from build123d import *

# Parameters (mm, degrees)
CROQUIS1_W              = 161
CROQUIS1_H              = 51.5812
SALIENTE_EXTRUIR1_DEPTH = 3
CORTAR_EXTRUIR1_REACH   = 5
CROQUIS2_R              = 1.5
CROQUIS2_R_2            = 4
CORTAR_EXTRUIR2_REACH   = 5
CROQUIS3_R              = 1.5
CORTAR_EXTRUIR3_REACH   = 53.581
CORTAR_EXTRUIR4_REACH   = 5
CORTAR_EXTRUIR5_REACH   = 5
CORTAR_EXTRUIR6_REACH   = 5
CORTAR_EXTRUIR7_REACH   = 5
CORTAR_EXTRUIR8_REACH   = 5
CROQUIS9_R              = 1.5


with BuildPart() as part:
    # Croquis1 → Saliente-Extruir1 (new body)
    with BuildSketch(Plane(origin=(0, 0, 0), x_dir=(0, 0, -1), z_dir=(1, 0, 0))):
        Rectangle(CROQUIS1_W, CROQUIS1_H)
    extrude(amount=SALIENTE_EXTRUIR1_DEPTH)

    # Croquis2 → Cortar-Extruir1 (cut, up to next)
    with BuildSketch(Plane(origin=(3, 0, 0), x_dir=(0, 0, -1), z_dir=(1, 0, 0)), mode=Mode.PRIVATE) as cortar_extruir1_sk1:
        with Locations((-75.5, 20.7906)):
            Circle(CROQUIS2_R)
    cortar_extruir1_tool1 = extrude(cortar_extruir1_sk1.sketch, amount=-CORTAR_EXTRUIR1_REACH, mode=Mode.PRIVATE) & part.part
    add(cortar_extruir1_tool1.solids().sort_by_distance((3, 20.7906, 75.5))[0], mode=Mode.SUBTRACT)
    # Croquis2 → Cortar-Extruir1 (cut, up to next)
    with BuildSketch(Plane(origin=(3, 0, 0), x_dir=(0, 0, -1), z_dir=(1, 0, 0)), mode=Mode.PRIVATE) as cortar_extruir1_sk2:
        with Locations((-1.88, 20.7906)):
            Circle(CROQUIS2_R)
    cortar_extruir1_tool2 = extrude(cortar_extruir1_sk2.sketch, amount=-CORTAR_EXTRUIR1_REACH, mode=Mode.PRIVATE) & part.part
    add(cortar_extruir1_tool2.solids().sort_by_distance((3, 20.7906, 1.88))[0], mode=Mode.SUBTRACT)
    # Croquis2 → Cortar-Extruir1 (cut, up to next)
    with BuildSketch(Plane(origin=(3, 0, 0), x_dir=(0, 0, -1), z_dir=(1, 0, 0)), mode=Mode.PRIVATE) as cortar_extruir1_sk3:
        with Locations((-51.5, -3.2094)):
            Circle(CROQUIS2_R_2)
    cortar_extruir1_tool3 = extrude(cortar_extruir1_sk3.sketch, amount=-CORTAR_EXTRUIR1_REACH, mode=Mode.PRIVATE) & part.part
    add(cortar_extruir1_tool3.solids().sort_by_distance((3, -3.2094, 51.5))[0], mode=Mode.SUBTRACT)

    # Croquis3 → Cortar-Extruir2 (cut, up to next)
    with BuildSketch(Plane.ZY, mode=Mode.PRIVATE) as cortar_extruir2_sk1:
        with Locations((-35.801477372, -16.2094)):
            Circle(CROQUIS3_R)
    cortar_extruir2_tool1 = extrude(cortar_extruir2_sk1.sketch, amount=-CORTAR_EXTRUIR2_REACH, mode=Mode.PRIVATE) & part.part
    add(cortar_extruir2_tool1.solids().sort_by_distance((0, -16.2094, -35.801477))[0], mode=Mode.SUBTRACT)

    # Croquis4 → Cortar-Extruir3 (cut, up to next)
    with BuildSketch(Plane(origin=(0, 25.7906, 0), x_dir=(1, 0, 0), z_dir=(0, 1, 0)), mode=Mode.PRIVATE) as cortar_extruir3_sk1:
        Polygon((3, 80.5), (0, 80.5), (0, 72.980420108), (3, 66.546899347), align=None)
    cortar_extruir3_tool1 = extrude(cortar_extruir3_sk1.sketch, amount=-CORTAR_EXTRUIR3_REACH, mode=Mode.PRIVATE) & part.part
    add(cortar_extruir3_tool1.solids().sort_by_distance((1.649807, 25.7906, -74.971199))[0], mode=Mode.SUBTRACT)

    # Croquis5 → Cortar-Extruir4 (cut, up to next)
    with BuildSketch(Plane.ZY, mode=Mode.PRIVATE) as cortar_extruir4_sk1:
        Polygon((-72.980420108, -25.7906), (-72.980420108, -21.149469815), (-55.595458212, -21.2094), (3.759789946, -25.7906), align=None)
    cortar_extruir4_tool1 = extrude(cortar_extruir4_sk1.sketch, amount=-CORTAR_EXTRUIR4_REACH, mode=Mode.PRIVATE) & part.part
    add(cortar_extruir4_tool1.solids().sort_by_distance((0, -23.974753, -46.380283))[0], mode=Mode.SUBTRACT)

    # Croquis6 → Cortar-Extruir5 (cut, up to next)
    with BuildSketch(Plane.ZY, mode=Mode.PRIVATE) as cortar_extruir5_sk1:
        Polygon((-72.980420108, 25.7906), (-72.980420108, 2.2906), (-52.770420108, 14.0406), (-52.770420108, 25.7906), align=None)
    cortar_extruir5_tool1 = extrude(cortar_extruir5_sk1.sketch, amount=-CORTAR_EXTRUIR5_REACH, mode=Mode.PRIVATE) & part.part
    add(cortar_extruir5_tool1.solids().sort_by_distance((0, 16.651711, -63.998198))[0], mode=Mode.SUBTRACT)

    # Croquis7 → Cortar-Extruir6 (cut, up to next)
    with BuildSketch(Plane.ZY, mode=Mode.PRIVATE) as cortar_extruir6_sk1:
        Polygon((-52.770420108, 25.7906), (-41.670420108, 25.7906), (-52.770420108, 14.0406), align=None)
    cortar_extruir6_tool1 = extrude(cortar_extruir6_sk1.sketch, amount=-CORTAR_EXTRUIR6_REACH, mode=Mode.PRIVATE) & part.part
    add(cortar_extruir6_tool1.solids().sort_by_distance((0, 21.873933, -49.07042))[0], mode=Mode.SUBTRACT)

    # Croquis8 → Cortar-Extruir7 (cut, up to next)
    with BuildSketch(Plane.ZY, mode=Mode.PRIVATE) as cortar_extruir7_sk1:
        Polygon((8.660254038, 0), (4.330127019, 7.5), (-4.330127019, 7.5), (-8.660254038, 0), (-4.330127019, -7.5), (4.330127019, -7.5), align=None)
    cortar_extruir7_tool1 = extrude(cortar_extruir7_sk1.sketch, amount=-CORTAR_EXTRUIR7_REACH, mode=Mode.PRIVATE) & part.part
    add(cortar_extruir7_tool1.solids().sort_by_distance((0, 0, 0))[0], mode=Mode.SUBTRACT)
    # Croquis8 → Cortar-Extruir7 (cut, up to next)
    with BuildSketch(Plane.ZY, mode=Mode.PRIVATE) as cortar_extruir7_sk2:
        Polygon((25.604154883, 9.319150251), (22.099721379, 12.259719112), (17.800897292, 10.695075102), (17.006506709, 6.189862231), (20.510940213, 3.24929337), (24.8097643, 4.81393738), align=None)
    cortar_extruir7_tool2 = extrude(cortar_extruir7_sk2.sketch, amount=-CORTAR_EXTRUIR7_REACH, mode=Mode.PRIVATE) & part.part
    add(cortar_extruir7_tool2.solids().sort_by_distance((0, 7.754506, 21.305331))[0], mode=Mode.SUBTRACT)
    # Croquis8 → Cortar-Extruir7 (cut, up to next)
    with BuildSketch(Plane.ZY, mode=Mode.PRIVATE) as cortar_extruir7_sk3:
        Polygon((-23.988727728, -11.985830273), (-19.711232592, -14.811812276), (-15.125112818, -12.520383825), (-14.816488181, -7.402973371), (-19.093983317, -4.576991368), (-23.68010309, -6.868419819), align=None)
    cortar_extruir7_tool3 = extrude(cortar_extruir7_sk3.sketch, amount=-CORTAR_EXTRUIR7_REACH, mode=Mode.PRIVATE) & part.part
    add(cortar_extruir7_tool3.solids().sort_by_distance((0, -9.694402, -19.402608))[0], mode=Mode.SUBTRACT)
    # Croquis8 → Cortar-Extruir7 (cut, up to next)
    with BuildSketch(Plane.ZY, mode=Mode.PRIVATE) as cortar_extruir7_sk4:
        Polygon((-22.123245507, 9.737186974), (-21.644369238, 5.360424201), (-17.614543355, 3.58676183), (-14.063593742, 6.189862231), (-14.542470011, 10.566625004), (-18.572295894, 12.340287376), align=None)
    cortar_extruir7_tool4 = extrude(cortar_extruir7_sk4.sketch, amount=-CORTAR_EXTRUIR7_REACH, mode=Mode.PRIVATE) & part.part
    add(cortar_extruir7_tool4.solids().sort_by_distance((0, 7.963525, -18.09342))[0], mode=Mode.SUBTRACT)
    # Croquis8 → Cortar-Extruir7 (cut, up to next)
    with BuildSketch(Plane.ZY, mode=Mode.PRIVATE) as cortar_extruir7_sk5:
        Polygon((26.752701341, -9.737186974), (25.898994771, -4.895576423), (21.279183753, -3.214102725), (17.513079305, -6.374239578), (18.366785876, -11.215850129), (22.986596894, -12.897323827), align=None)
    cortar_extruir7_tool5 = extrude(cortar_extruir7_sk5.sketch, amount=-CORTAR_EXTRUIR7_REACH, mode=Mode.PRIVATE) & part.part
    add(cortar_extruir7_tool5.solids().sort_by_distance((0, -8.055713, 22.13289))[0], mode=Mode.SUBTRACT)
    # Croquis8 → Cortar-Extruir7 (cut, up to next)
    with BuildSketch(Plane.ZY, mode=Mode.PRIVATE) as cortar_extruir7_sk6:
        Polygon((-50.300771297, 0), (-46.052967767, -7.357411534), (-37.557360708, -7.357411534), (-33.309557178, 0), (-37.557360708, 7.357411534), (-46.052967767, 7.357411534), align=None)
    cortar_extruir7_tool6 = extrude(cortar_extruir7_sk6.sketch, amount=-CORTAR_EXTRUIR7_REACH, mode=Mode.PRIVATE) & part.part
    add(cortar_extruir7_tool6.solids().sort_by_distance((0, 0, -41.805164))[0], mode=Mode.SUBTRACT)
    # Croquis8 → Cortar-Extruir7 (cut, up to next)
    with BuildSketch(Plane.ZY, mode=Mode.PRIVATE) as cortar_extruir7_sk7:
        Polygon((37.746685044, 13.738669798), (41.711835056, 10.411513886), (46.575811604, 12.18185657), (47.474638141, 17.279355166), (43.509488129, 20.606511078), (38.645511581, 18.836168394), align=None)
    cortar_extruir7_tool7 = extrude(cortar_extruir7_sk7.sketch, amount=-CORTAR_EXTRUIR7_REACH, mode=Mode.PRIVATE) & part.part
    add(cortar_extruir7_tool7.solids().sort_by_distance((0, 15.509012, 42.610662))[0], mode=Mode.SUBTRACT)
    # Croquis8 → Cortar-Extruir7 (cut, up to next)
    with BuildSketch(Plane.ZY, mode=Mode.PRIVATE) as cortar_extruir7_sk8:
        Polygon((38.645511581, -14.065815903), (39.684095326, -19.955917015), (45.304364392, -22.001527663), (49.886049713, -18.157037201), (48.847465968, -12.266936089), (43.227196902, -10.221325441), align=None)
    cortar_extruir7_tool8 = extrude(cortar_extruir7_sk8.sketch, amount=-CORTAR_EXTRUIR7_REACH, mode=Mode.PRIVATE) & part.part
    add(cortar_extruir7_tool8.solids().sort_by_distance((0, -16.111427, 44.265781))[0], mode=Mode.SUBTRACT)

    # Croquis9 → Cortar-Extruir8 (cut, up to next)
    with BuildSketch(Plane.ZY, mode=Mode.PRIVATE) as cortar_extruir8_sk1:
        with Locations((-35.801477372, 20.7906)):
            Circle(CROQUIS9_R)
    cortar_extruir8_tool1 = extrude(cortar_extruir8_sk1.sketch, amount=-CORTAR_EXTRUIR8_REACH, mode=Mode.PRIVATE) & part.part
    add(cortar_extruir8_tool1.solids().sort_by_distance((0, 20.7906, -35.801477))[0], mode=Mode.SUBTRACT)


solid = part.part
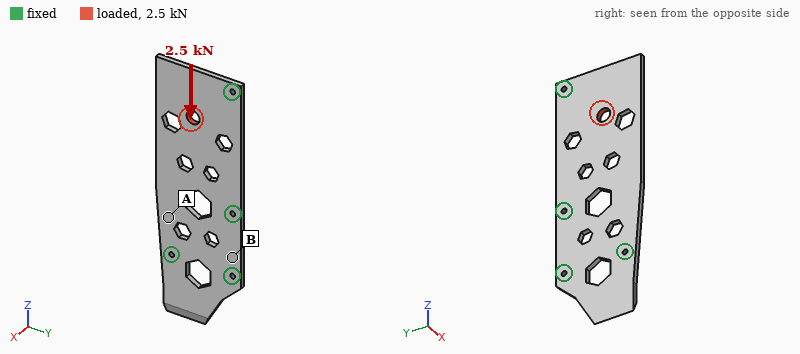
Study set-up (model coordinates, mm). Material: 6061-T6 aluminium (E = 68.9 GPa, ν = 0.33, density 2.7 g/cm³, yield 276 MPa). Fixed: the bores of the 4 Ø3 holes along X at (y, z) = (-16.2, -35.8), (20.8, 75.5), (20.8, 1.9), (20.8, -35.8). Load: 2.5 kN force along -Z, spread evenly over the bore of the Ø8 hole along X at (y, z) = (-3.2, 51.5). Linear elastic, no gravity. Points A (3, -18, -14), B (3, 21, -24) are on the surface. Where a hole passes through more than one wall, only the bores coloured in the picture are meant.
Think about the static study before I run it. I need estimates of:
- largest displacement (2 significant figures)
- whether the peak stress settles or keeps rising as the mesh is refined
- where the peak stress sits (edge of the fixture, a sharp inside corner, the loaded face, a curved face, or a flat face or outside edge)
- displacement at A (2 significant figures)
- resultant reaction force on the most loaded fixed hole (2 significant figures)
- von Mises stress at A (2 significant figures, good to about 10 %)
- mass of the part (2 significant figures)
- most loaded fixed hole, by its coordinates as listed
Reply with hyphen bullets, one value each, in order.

- 22 µm
- keeps rising
- edge of the fixture
- 4.3 µm
- 1.1 kN
- 13 MPa
- 51 g
- (20.8, 75.5)
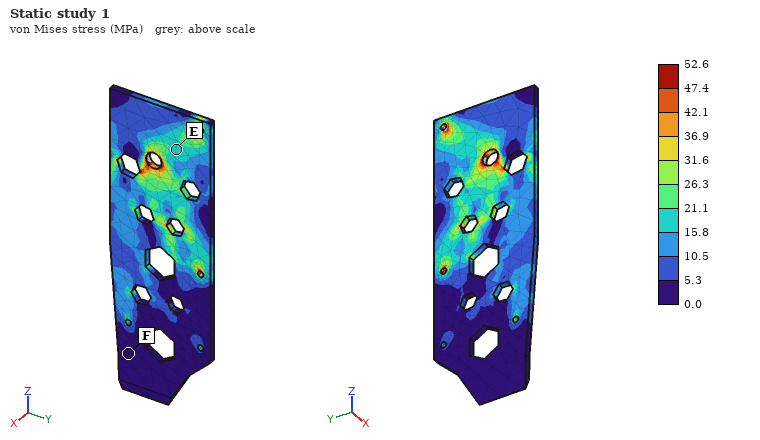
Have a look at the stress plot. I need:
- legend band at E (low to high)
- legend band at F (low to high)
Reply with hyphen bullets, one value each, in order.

- 15.8 to 21.1 MPa
- 0.0 to 5.3 MPa
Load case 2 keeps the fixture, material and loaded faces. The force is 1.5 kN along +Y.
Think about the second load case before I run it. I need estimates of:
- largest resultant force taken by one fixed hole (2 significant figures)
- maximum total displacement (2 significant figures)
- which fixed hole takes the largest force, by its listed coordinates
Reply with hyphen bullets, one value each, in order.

- 1.1 kN
- 17 µm
- (20.8, 75.5)
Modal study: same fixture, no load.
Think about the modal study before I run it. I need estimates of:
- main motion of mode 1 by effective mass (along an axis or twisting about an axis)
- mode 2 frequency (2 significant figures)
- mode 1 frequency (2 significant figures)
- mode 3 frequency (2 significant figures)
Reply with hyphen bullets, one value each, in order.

- along X
- 2000 Hz
- 930 Hz
- 2000 Hz
